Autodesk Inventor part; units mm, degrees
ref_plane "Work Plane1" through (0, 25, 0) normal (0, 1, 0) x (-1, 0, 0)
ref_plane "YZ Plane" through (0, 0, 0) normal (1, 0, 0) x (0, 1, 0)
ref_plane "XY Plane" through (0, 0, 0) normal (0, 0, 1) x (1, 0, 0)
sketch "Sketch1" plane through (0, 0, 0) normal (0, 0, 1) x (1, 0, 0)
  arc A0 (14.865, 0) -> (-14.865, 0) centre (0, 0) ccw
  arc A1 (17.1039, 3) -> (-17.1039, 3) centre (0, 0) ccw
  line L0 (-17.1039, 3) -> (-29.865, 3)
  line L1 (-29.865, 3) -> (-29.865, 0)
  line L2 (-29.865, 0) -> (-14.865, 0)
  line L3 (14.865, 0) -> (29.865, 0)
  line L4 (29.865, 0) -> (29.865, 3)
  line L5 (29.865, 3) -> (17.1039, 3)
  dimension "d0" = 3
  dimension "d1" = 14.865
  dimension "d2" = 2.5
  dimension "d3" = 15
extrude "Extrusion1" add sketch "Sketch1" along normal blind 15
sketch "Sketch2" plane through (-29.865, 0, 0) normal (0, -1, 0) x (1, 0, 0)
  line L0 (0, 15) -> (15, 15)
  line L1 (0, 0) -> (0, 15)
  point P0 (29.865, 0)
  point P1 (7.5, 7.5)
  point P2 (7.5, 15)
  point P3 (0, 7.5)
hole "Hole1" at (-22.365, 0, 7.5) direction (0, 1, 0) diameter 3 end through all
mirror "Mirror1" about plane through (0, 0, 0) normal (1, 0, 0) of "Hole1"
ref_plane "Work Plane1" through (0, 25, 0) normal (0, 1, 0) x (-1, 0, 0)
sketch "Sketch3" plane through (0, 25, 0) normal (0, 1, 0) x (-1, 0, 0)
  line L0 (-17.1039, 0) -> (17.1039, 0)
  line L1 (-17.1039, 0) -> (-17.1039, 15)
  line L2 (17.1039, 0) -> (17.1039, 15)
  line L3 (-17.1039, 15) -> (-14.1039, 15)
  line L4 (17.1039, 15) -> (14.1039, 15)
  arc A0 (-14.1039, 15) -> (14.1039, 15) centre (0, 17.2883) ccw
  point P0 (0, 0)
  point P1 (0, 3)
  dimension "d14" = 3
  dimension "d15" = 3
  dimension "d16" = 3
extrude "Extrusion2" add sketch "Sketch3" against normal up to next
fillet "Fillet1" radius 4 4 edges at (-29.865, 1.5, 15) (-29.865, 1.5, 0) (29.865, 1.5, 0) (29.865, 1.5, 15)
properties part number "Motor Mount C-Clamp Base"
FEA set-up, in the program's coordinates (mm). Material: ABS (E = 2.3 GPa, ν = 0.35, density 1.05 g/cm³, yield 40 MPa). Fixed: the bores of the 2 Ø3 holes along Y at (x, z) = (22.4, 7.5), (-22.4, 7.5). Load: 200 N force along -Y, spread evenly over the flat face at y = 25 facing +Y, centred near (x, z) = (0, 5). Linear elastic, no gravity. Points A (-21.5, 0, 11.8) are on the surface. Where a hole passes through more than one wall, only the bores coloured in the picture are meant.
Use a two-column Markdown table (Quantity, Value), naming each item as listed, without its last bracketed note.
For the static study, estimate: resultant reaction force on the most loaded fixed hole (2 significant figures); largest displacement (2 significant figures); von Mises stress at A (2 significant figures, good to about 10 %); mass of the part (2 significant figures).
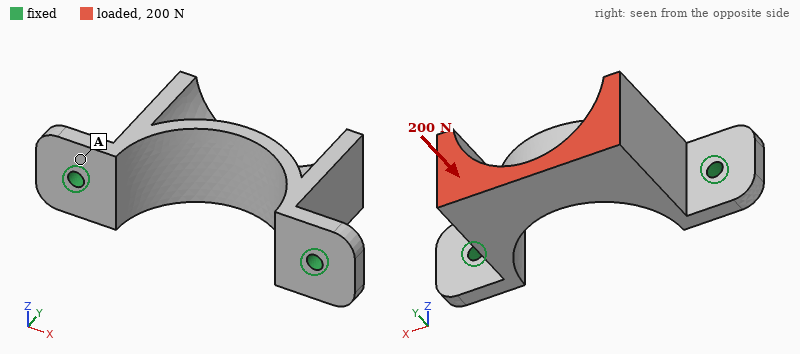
| Quantity | Value |
|---|---|
| resultant reaction force on the most loaded fixed hole | 110 N |
| largest displacement | 0.35 mm |
| von Mises stress at A | 4.4 MPa |
| mass of the part | 6.7 g |
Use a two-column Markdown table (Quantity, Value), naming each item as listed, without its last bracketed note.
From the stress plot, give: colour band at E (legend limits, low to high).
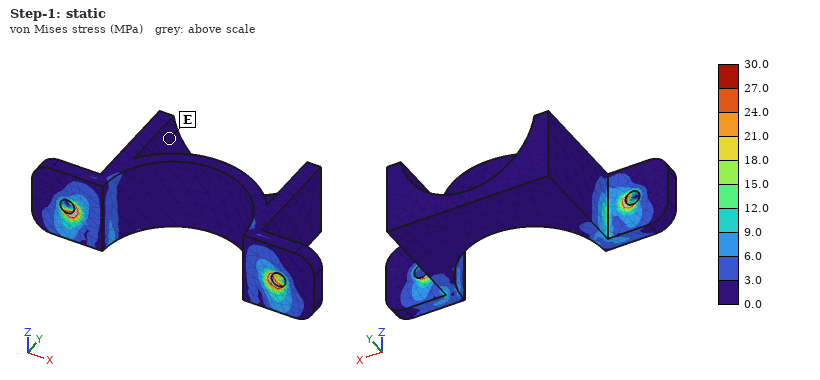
| Quantity | Value |
|---|---|
| colour band at E | 0.0 to 3.0 MPa |
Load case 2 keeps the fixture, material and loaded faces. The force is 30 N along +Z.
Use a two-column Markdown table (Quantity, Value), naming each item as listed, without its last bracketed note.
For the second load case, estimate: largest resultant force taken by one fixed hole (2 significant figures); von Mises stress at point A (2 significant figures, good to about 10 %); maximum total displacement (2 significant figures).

| Quantity | Value |
|---|---|
| largest resultant force taken by one fixed hole | 15 N |
| von Mises stress at point A | 7.8 MPa |
| maximum total displacement | 0.45 mm |
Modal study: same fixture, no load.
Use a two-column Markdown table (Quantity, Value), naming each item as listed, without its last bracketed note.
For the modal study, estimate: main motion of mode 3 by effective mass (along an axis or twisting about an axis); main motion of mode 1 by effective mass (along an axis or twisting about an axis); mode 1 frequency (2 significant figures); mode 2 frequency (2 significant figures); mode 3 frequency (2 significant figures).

| Quantity | Value |
|---|---|
| main motion of mode 3 by effective mass | along X |
| main motion of mode 1 by effective mass | along Z |
| mode 1 frequency | 840 Hz |
| mode 2 frequency | 1800 Hz |
| mode 3 frequency | 2900 Hz |
